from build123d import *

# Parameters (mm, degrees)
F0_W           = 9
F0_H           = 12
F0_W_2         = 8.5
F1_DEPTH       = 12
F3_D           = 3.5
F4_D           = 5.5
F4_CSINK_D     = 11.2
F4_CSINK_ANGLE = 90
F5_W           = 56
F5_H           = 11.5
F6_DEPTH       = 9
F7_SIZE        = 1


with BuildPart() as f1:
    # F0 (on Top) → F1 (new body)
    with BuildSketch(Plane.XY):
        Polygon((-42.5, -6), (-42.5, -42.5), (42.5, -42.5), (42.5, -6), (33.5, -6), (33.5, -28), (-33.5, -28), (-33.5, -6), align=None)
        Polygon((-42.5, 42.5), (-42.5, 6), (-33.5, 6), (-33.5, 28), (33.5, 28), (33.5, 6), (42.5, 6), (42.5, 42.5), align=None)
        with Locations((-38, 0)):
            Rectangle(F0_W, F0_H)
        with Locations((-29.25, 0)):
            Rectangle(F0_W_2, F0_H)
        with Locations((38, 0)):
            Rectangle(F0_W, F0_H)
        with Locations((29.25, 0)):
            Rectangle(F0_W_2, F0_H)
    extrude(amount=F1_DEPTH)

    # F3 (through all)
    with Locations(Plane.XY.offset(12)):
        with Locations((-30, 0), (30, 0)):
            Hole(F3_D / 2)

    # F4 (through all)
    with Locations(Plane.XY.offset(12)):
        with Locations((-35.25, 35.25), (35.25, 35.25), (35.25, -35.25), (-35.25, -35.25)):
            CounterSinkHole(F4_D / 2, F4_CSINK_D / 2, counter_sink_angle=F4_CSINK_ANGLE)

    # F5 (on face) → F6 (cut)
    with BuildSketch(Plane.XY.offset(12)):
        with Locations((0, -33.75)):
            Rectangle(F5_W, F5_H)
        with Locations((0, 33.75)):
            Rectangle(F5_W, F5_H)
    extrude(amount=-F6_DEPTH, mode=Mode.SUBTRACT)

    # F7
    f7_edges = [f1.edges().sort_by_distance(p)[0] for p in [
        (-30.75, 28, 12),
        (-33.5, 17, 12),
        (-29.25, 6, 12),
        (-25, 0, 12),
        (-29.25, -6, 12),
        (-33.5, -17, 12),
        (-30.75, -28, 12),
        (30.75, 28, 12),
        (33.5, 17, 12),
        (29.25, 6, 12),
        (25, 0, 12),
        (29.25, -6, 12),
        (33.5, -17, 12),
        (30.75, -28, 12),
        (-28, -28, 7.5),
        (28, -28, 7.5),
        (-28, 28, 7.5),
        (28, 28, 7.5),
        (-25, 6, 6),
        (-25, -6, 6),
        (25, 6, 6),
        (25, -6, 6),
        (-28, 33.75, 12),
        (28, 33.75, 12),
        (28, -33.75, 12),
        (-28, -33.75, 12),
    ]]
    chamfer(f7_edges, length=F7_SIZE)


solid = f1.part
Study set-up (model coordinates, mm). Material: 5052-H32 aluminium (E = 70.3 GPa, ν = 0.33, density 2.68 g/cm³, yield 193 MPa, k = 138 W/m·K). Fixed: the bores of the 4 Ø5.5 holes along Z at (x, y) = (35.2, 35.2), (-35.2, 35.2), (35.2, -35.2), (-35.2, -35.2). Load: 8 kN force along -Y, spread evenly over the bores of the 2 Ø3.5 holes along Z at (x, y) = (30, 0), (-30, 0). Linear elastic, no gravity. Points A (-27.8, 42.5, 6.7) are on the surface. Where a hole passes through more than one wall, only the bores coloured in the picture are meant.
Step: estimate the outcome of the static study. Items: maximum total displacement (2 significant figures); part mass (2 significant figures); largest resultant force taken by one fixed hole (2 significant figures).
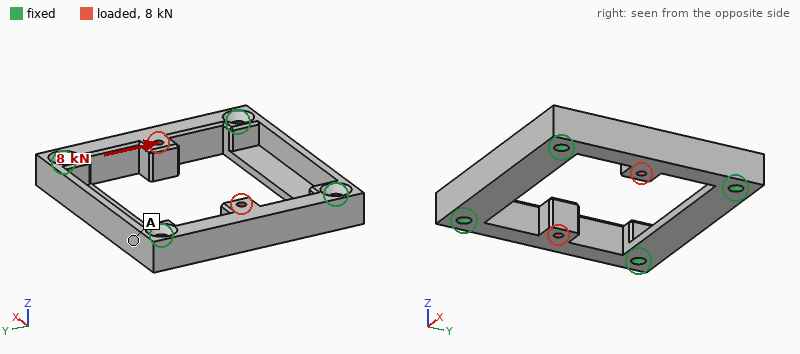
49 µm
82 g
2.1 kN
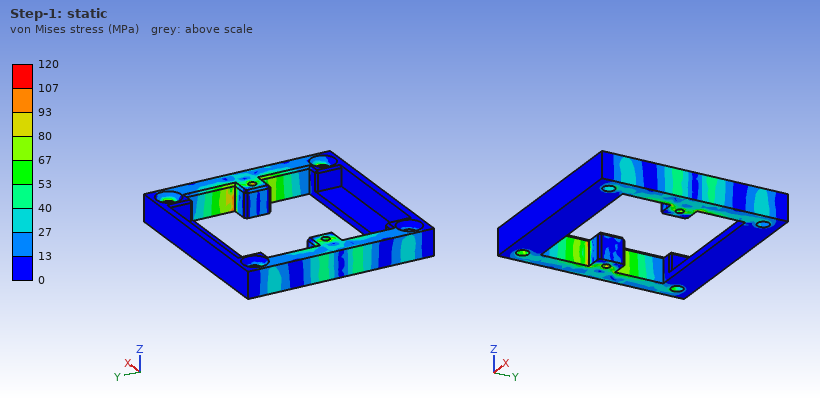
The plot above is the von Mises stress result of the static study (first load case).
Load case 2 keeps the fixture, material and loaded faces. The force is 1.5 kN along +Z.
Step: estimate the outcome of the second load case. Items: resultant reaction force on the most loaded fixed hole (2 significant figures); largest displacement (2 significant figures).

380 N
49 µm
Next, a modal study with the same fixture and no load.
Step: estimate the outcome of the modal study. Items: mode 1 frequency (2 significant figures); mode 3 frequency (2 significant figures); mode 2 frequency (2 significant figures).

7700 Hz
8300 Hz
7700 Hz
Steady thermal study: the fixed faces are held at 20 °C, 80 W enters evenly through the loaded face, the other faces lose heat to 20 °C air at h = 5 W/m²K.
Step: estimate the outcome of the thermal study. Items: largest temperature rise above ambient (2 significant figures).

56 K
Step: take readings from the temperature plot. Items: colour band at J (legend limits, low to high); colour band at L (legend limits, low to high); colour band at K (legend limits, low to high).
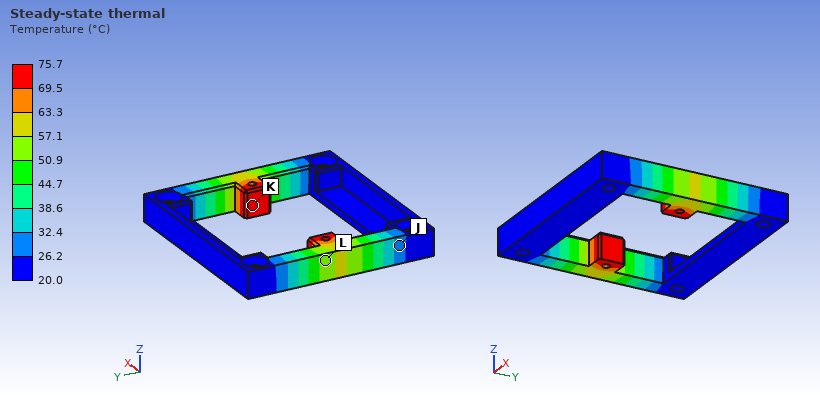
26.2 to 32.4 °C
50.9 to 57.1 °C
69.5 to 75.7 °C
